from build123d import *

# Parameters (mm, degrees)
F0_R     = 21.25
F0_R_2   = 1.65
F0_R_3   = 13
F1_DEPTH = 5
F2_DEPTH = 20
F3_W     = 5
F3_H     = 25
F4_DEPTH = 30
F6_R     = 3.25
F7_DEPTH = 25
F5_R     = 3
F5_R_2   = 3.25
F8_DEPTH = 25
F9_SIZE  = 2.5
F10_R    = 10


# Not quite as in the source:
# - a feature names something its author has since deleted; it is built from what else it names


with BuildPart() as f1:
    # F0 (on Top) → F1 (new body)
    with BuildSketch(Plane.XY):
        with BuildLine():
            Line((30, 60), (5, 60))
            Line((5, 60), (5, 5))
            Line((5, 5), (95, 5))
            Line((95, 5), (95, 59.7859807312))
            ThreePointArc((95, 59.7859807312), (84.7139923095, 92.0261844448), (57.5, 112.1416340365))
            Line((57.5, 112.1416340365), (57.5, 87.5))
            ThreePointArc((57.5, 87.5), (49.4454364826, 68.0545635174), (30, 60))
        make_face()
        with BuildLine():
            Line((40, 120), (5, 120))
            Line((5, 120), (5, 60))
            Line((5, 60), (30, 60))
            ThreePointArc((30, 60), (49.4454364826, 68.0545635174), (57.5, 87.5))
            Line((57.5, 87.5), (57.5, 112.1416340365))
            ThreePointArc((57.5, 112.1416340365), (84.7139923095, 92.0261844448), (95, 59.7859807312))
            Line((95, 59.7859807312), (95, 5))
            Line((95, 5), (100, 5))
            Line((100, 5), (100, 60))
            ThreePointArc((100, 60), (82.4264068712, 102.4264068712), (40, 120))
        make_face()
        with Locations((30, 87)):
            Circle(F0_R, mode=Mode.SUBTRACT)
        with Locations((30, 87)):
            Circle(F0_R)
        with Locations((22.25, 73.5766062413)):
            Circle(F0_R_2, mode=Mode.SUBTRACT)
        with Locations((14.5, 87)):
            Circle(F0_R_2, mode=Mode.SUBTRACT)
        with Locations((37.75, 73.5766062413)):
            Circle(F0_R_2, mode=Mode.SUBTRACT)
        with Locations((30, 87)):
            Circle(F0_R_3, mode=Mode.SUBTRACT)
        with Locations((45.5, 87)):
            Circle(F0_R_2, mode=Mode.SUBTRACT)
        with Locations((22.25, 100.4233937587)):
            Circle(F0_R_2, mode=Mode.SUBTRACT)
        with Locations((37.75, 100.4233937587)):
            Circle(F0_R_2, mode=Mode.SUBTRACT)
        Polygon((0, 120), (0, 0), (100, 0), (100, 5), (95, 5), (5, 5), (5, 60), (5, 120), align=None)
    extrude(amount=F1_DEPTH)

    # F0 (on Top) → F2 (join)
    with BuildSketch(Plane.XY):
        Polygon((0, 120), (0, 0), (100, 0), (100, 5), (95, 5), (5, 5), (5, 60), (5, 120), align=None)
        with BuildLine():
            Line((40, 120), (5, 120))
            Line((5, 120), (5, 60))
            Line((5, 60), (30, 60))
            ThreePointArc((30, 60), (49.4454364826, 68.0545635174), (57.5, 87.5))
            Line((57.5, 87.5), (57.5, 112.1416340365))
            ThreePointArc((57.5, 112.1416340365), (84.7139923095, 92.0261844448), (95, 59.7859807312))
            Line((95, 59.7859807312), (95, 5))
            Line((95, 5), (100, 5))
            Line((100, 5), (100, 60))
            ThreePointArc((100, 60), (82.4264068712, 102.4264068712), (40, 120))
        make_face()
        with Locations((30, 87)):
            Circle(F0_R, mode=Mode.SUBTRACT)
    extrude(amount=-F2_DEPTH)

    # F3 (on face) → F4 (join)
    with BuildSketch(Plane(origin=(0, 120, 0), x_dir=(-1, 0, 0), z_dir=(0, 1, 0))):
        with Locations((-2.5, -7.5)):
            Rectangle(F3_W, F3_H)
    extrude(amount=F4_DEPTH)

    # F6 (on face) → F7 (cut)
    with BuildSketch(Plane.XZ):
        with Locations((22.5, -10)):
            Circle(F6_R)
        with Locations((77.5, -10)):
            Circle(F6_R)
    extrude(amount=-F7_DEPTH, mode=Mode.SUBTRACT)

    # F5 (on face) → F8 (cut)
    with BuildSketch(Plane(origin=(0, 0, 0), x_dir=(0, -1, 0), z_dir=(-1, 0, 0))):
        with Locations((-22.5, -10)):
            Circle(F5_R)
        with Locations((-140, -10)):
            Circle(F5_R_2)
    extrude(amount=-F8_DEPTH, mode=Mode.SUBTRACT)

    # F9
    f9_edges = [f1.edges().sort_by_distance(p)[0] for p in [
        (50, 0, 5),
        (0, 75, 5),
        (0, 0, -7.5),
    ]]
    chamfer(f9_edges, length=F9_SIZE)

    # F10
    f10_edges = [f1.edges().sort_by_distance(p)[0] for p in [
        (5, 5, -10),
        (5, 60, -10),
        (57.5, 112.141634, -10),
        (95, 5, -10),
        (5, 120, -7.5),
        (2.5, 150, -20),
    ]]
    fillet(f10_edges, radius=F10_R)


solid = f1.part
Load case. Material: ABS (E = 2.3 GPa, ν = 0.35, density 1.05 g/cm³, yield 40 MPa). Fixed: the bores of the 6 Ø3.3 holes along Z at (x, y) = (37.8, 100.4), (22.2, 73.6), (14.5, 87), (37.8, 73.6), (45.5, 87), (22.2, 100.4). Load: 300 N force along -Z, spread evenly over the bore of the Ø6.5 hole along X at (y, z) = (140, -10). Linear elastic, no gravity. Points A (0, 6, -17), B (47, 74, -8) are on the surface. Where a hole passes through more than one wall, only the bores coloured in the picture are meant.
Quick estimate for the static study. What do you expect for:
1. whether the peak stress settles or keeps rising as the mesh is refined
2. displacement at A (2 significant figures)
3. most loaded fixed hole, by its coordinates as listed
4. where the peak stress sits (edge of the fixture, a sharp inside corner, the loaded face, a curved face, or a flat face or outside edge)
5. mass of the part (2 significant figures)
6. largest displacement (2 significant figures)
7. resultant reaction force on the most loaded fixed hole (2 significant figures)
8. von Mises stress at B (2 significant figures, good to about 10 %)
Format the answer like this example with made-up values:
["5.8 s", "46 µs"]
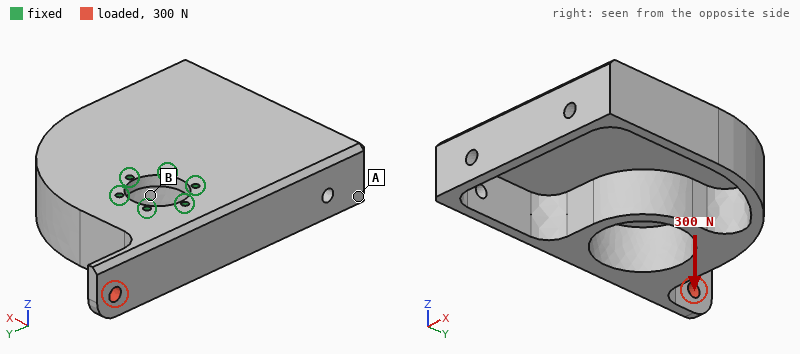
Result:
["keeps rising", "0.47 mm", "(22.2, 100.4)", "edge of the fixture", "130 g", "1.0 mm", "470 N", "2.6 MPa"]
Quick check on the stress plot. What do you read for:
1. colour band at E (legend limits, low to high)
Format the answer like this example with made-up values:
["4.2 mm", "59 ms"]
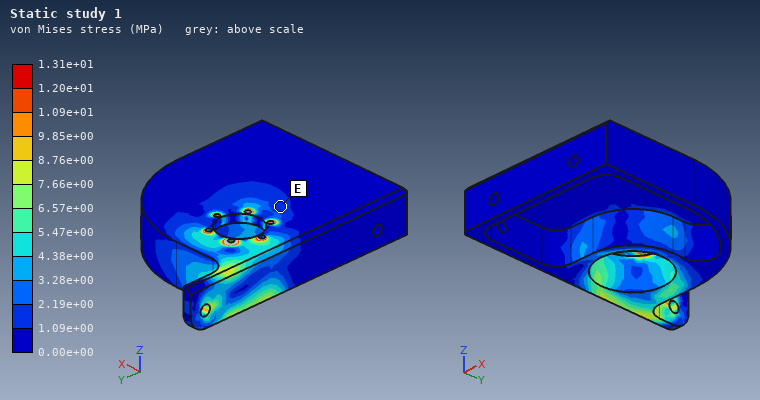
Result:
["1.09e+00 to 2.19e+00 MPa"]
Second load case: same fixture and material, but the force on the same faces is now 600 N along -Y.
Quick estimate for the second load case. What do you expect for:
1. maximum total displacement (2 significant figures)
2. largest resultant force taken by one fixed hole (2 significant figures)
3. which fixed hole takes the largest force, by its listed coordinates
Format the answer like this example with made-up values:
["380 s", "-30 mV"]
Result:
["0.46 mm", "390 N", "(14.5, 87)"]
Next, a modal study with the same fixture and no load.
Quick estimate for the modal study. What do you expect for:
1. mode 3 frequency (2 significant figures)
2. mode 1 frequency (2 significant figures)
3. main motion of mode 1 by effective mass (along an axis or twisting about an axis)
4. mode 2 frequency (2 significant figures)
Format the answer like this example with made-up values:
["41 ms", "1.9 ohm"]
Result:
["840 Hz", "250 Hz", "along Z", "510 Hz"]
